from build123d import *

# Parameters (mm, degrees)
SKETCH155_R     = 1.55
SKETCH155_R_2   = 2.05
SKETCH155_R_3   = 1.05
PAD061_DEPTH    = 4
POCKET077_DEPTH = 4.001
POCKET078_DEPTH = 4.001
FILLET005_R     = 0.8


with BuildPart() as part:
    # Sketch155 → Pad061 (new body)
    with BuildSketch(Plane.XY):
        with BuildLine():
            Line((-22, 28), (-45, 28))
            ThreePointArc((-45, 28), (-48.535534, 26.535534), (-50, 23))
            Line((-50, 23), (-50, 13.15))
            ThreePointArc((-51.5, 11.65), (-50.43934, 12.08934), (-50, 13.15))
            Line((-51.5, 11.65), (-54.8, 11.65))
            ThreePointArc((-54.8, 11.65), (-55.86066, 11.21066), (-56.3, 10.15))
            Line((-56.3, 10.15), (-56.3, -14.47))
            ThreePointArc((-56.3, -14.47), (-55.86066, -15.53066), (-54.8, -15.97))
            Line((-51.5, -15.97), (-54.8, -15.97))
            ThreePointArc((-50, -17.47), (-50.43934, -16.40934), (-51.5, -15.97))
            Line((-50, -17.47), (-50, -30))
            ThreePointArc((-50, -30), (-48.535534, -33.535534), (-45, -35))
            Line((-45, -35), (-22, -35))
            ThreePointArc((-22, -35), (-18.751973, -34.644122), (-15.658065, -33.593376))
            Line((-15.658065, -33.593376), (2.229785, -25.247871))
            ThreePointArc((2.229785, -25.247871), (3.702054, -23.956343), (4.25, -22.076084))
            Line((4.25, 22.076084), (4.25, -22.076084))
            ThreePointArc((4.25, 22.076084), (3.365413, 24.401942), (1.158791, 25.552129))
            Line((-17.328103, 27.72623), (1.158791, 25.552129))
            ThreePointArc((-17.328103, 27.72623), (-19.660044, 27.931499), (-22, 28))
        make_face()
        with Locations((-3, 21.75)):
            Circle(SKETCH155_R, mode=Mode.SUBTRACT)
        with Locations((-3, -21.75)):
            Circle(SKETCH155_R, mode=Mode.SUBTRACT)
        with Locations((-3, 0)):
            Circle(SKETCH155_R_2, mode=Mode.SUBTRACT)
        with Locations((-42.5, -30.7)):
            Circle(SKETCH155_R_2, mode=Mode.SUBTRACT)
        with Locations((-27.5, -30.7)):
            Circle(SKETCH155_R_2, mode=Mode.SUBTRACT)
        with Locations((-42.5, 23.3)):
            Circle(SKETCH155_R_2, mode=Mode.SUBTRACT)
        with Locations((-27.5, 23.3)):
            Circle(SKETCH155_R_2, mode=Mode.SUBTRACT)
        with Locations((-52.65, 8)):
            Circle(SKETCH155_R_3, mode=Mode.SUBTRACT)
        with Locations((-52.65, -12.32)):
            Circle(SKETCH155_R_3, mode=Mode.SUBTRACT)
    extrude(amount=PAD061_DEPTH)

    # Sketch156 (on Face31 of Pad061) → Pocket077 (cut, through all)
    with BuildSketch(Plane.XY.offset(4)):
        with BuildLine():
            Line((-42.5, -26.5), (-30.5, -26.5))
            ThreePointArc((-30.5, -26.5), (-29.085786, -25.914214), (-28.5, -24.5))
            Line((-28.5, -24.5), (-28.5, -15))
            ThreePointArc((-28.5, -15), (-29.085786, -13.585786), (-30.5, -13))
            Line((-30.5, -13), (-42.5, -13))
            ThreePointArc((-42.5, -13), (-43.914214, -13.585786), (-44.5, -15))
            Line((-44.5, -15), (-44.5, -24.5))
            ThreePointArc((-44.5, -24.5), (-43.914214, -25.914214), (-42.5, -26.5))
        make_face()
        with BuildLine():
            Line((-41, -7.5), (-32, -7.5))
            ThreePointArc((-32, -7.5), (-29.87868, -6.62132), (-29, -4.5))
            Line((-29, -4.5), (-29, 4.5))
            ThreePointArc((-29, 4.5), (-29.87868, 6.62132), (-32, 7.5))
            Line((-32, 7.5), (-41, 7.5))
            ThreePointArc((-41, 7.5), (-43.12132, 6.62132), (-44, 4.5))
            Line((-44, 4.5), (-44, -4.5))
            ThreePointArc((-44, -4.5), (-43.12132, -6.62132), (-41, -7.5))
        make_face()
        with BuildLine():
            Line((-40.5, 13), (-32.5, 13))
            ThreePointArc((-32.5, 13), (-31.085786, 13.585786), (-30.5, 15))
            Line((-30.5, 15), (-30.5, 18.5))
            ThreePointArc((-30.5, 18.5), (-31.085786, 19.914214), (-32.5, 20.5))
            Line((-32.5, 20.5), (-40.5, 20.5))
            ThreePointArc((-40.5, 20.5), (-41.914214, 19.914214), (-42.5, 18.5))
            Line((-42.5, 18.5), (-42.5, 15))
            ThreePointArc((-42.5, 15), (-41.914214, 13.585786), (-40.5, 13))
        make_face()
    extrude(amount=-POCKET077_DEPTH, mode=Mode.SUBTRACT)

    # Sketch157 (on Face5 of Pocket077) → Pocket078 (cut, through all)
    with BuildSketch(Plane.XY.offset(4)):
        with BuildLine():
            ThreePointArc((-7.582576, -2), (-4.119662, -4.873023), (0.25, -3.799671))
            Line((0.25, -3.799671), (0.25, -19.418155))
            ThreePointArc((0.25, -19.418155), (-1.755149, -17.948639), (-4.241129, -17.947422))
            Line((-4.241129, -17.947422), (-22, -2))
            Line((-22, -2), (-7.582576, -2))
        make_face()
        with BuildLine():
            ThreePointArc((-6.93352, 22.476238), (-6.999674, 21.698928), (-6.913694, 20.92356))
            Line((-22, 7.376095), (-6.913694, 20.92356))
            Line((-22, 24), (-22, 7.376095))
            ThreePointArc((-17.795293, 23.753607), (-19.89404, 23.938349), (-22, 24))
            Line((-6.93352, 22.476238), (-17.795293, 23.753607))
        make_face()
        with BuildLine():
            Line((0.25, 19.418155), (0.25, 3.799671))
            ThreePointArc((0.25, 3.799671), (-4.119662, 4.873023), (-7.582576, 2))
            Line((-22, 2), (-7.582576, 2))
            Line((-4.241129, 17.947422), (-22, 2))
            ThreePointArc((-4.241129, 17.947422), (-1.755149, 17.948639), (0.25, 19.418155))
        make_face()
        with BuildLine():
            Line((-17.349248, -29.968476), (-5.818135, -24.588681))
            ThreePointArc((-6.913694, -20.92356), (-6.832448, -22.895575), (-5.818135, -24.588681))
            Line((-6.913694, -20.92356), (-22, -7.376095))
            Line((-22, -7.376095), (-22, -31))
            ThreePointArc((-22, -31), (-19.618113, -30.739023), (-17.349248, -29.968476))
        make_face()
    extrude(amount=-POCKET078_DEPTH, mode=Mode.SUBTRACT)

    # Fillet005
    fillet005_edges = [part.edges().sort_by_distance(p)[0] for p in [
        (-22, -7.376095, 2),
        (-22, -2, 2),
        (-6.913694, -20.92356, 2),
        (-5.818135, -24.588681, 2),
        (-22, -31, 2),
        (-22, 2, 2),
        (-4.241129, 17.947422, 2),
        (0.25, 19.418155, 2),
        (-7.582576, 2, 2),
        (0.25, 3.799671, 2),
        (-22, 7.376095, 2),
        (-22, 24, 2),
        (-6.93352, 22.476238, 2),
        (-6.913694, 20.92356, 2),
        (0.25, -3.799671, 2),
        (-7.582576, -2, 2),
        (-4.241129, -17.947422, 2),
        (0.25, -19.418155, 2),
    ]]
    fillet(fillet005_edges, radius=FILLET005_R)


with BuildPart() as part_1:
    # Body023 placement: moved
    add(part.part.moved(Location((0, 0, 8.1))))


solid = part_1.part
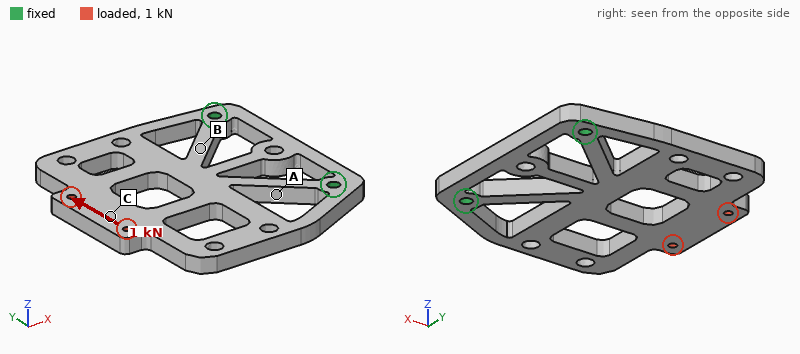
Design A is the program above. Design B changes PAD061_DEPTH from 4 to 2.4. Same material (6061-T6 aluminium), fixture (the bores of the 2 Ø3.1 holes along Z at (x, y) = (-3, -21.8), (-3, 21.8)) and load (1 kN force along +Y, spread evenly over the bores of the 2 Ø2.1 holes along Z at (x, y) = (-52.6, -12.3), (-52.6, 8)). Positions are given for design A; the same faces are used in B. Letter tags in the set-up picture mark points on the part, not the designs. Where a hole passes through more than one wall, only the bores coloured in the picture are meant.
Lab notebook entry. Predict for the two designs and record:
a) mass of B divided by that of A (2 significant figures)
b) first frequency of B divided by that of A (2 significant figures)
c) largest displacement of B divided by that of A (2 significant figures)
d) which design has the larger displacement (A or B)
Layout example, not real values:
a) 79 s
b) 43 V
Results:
a) 0.60
b) 0.63
c) 1.7
d) B
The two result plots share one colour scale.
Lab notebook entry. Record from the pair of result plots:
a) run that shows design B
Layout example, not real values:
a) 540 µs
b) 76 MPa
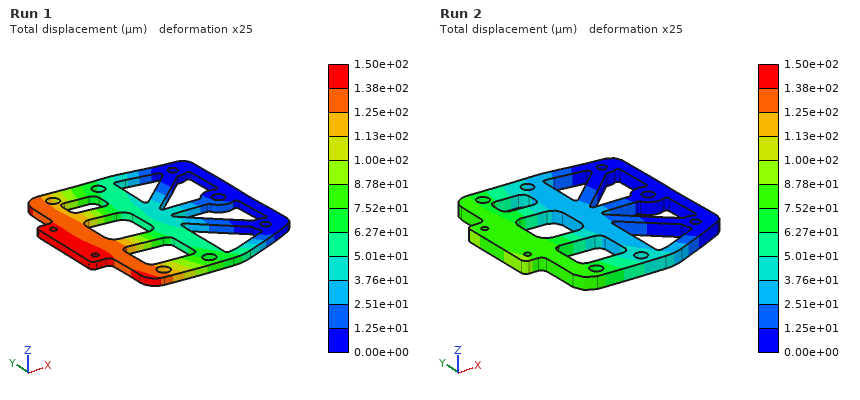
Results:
a) Run 1
